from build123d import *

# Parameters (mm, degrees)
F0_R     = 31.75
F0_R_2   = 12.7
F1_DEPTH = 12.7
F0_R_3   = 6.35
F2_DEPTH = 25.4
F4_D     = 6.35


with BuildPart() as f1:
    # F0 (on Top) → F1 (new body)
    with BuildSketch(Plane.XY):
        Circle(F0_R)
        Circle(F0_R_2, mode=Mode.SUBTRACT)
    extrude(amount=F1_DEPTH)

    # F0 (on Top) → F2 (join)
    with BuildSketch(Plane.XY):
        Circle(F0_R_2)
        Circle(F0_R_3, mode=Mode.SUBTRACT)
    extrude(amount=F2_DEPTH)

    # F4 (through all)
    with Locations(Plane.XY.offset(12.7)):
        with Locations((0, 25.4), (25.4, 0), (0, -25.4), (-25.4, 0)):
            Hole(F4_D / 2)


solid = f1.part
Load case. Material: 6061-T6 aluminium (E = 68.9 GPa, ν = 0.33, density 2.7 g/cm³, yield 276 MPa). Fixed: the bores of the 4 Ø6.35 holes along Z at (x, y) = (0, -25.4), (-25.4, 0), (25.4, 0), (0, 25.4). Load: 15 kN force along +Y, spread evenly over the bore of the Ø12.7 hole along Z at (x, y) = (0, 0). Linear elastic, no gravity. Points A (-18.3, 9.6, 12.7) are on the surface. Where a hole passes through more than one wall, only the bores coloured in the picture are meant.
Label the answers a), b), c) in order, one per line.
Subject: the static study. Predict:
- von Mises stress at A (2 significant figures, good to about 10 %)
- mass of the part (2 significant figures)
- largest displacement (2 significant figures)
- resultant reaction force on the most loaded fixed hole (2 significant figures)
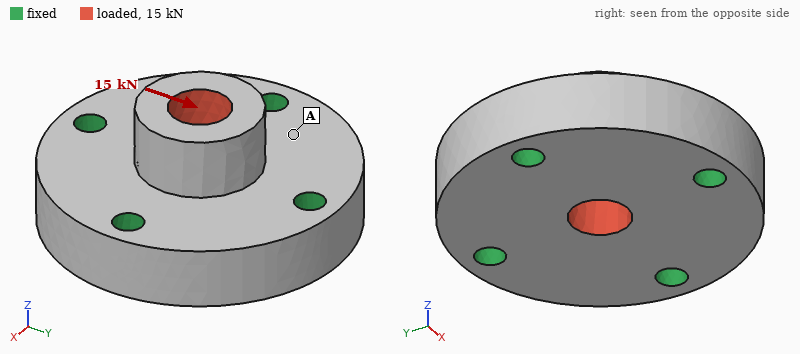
a) 8.4 MPa
b) 110 g
c) 25 µm
d) 5.3 kN
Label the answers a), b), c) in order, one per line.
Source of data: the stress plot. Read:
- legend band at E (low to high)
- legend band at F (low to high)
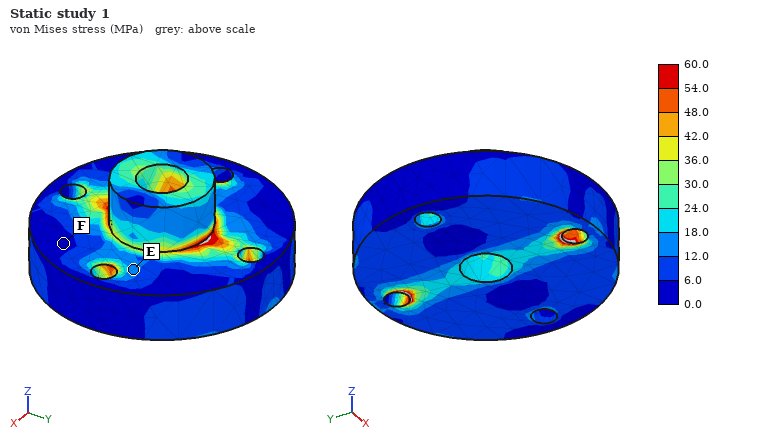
a) 12.0 to 18.0 MPa
b) 0.0 to 6.0 MPa
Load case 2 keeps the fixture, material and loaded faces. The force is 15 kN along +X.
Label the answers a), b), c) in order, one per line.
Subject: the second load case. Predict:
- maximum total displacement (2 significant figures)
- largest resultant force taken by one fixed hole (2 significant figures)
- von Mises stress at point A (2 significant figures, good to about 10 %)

a) 25 µm
b) 5.3 kN
c) 14 MPa
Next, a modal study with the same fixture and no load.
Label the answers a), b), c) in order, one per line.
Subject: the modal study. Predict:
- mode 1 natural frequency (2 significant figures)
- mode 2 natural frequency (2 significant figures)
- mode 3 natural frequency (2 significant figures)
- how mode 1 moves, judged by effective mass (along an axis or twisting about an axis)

a) 24 kHz
b) 26 kHz
c) 26 kHz
d) along Z
